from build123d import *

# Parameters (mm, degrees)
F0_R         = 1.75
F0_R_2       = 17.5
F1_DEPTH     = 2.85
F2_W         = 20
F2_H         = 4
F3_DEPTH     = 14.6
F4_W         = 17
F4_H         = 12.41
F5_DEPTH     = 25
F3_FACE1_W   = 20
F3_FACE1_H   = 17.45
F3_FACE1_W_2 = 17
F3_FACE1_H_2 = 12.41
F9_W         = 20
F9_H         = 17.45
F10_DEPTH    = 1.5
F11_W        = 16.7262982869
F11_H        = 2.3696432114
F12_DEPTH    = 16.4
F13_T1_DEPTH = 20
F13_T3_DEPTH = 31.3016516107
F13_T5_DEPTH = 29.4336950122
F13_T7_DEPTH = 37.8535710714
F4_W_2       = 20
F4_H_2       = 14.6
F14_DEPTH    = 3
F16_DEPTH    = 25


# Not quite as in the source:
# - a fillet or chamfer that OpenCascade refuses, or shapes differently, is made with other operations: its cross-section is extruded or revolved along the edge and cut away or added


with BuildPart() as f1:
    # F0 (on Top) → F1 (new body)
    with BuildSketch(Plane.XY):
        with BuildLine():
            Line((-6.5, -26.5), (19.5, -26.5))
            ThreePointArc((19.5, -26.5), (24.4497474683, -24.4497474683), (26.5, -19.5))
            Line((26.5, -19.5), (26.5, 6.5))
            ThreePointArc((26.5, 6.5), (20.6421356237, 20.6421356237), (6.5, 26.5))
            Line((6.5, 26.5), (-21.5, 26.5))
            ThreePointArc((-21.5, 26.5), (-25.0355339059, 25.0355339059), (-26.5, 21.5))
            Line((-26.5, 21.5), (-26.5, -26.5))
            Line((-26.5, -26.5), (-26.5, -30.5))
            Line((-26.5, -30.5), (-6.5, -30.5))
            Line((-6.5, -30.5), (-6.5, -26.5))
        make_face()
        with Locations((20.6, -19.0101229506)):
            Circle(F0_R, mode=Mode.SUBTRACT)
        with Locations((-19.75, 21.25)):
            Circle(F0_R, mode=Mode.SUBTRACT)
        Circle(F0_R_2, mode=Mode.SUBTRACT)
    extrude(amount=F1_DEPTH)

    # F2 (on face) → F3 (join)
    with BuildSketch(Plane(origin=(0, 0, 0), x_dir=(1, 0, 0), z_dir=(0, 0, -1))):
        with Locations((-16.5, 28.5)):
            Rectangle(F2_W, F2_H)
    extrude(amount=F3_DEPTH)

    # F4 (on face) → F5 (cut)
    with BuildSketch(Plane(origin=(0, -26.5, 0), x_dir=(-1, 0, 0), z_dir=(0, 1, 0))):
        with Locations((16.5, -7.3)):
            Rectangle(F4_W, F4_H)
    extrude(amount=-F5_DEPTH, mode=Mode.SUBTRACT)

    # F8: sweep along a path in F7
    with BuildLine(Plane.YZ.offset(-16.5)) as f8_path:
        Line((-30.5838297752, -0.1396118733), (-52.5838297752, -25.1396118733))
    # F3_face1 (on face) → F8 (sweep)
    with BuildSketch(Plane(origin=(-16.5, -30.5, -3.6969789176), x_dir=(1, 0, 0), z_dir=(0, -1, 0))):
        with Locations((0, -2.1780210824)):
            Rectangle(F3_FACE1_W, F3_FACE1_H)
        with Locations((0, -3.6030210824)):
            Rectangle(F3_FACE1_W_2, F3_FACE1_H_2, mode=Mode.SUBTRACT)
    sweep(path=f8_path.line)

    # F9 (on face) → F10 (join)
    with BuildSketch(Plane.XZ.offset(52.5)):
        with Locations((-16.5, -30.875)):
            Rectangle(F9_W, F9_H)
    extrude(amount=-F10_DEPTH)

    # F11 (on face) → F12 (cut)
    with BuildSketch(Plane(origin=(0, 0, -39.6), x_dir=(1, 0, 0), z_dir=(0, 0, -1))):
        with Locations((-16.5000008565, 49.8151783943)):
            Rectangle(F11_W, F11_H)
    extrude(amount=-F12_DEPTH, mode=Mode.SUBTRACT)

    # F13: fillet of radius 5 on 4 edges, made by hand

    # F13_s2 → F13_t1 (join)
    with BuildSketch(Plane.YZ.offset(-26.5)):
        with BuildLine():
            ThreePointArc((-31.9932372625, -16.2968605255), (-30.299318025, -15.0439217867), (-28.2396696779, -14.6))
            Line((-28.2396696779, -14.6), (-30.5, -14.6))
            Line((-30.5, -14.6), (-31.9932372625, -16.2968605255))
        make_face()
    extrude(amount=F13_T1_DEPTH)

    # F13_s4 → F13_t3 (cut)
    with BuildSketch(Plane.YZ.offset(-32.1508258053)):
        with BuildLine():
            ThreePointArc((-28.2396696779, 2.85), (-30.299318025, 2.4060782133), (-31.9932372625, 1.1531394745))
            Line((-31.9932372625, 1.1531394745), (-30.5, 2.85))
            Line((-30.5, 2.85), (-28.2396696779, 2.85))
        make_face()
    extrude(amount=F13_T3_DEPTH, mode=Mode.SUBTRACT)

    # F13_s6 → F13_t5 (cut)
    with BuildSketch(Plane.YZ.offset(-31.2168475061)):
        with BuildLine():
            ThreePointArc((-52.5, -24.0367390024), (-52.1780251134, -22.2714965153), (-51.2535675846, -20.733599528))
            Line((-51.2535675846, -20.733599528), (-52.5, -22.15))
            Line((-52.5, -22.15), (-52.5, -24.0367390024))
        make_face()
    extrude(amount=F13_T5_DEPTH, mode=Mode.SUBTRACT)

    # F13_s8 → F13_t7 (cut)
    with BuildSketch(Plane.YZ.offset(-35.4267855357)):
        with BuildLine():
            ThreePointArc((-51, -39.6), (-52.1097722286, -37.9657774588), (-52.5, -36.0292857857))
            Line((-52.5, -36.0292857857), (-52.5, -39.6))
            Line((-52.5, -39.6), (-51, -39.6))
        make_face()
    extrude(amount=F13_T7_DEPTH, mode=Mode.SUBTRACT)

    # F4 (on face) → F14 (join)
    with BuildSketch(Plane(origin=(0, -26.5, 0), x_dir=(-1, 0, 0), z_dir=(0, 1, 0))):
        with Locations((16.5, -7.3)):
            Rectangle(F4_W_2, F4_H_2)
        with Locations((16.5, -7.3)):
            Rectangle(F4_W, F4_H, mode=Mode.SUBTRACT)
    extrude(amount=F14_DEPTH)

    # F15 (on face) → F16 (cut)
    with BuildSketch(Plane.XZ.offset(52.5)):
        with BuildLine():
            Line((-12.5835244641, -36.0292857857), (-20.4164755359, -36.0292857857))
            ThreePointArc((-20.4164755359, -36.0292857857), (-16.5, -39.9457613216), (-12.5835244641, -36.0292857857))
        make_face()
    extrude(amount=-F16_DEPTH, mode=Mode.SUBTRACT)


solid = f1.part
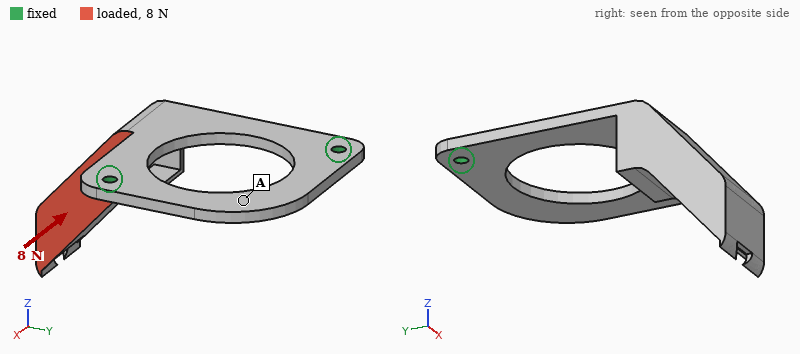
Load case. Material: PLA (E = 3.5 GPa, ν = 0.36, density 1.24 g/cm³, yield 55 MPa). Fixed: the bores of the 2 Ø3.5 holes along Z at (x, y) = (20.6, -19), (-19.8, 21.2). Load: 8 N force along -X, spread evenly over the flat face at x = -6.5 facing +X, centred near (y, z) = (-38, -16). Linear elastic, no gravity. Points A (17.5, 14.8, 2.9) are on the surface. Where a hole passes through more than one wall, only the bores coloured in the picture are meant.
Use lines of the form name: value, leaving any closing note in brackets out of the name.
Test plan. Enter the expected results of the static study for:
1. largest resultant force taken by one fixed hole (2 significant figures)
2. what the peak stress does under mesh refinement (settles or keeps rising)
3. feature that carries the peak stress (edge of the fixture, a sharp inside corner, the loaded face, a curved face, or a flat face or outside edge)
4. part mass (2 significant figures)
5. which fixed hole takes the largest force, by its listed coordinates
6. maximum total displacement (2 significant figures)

largest resultant force taken by one fixed hole: 9.7 N
what the peak stress does under mesh refinement: keeps rising
feature that carries the peak stress: edge of the fixture
part mass: 11 g
which fixed hole takes the largest force, by its listed coordinates: (20.6, -19)
maximum total displacement: 1.2 mm
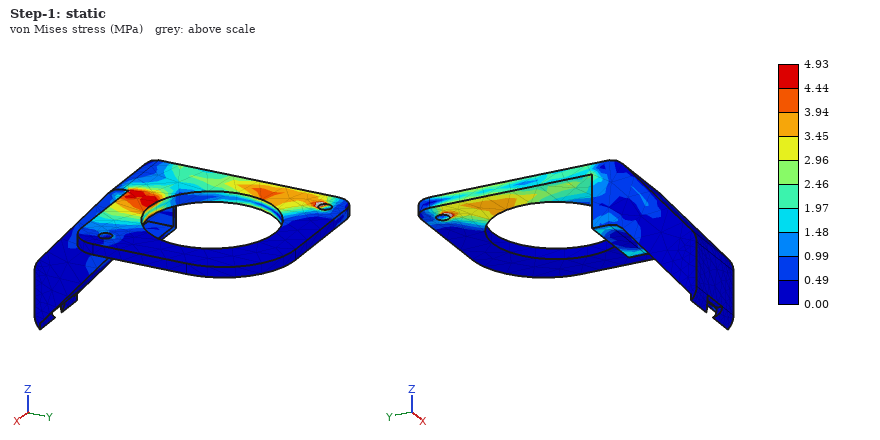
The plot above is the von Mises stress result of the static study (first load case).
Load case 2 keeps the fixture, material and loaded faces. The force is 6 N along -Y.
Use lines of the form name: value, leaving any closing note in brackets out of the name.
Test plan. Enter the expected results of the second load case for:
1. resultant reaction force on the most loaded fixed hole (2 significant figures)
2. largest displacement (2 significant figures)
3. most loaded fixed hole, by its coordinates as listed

resultant reaction force on the most loaded fixed hole: 4.3 N
largest displacement: 1.1 mm
most loaded fixed hole, by its coordinates as listed: (-19.8, 21.2)
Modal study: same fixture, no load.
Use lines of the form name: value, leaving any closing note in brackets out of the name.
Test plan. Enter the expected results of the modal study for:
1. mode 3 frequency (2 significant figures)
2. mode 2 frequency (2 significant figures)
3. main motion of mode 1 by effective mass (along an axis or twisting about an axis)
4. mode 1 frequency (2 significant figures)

mode 3 frequency: 670 Hz
mode 2 frequency: 360 Hz
main motion of mode 1 by effective mass: along Z
mode 1 frequency: 140 Hz
